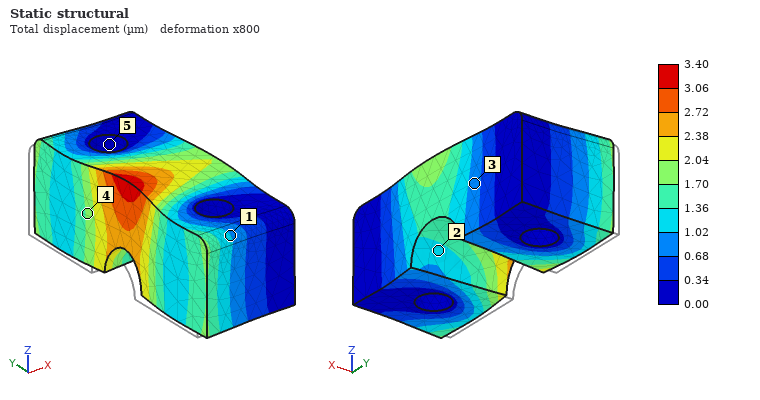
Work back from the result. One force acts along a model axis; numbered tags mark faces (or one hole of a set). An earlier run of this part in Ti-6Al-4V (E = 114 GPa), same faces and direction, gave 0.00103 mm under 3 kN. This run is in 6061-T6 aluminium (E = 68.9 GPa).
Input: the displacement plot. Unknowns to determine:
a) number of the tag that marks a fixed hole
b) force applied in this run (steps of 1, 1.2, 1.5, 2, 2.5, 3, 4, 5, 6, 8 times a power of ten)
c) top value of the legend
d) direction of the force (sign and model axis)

5
6 kN
3.40 µm
+X
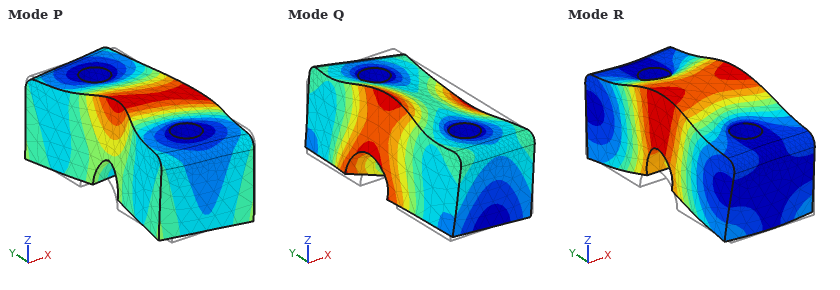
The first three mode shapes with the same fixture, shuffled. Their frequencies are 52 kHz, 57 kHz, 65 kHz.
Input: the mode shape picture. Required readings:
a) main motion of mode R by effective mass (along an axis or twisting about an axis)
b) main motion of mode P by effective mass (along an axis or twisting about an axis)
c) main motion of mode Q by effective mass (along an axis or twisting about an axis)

along Z
along X
twisting about Y
